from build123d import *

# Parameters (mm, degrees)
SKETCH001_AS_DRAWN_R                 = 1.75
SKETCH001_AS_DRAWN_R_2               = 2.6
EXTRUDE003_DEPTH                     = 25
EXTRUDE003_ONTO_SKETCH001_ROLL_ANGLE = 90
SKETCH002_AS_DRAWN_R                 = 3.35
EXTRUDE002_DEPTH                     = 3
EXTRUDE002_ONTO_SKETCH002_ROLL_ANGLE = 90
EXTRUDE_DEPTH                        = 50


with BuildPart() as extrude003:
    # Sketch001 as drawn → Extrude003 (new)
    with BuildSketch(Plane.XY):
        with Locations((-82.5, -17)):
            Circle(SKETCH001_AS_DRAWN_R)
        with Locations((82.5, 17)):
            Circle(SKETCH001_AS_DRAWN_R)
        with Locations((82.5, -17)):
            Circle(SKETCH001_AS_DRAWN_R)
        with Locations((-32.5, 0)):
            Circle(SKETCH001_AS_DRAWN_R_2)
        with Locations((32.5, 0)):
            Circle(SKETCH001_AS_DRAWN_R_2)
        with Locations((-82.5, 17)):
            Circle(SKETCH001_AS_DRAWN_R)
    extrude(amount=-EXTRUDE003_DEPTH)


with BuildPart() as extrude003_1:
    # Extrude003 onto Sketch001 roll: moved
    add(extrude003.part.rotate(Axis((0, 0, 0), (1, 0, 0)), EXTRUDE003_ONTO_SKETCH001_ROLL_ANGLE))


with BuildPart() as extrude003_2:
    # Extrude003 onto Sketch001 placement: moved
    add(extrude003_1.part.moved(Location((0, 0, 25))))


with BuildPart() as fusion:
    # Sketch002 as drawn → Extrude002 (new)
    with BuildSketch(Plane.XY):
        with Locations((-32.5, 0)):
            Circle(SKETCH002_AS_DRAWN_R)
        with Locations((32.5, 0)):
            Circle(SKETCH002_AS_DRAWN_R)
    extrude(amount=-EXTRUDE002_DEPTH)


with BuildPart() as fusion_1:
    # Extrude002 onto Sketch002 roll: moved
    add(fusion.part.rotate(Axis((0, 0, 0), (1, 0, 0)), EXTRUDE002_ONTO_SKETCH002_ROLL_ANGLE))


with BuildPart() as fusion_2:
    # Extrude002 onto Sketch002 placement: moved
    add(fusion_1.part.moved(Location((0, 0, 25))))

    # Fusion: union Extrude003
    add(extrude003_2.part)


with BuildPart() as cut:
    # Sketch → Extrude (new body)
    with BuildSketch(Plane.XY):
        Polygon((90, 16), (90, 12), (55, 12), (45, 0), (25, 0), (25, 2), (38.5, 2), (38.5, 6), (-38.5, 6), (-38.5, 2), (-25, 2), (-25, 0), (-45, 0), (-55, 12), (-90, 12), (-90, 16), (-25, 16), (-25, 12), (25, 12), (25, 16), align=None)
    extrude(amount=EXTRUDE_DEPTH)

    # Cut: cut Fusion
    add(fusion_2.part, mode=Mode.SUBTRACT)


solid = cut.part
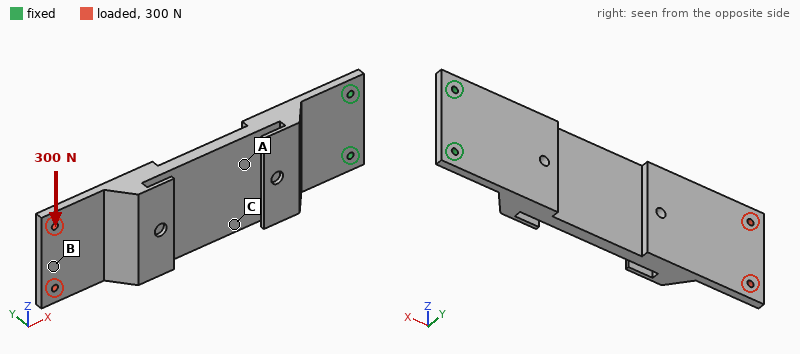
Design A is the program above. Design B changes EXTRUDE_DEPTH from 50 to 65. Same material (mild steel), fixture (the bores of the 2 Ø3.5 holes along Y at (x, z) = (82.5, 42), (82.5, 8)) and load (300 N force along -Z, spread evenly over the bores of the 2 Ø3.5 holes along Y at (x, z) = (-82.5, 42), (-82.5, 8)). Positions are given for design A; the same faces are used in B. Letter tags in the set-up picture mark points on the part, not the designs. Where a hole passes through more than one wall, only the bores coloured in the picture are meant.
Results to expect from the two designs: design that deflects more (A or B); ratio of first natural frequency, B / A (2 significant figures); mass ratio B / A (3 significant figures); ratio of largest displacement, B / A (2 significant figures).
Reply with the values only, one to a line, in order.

A
0.97
1.30
0.72
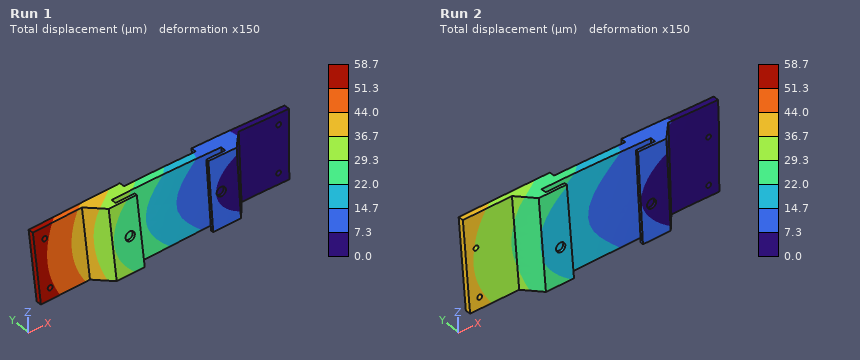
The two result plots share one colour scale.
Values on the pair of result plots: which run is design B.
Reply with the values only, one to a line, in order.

Run 2
